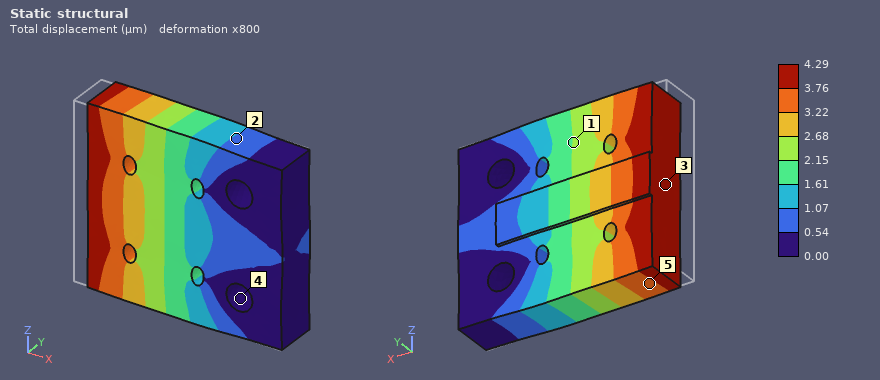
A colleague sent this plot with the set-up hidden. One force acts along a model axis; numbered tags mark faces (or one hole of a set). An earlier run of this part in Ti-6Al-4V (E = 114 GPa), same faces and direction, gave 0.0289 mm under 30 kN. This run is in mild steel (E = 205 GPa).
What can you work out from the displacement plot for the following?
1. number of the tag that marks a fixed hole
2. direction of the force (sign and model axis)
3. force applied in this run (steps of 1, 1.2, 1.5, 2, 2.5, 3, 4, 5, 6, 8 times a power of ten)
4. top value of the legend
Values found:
4
+X
8 kN
4.29 µm
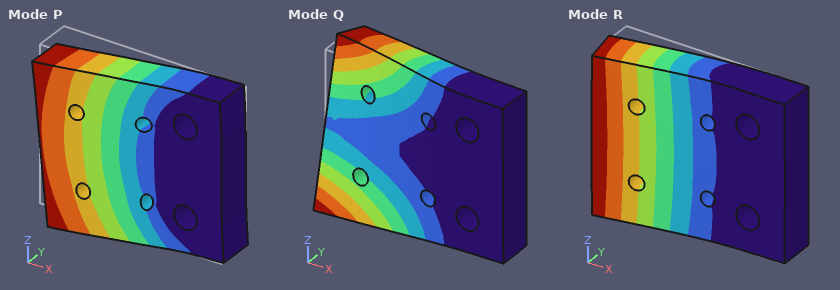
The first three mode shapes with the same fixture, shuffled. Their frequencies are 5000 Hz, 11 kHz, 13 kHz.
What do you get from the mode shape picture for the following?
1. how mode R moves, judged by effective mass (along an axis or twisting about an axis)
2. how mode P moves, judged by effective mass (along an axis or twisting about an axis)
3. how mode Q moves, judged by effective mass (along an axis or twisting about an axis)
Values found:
along Y
along Z
twisting about X
